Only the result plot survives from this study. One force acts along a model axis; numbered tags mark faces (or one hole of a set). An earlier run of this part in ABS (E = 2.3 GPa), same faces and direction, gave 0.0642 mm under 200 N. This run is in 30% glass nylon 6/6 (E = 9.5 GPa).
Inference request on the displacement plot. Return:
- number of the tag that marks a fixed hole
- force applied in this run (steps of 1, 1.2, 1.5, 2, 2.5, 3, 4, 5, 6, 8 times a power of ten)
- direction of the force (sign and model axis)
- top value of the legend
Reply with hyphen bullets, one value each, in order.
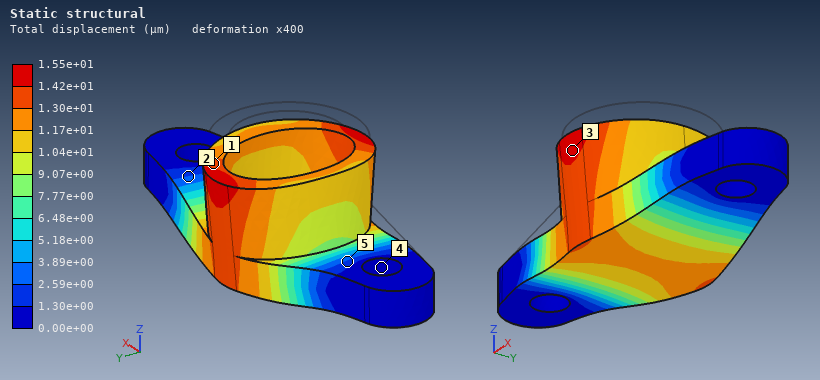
- 4
- 200 N
- -Z
- 1.55e+01 µm
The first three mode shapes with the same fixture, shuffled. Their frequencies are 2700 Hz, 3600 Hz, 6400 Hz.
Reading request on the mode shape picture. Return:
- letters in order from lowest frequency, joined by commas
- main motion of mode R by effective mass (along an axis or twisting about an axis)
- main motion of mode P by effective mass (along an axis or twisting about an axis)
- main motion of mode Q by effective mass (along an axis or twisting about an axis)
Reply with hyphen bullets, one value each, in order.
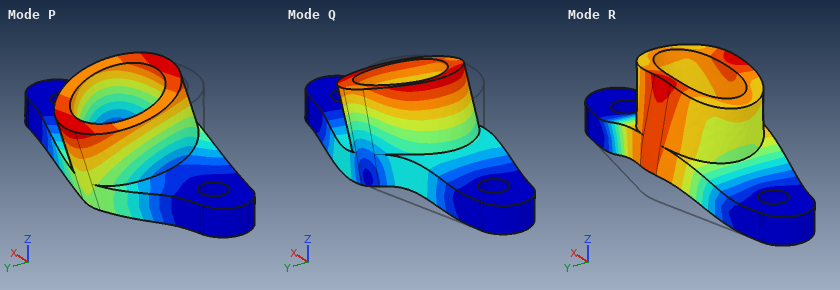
- P, R, Q
- along Z
- along Y
- along X
